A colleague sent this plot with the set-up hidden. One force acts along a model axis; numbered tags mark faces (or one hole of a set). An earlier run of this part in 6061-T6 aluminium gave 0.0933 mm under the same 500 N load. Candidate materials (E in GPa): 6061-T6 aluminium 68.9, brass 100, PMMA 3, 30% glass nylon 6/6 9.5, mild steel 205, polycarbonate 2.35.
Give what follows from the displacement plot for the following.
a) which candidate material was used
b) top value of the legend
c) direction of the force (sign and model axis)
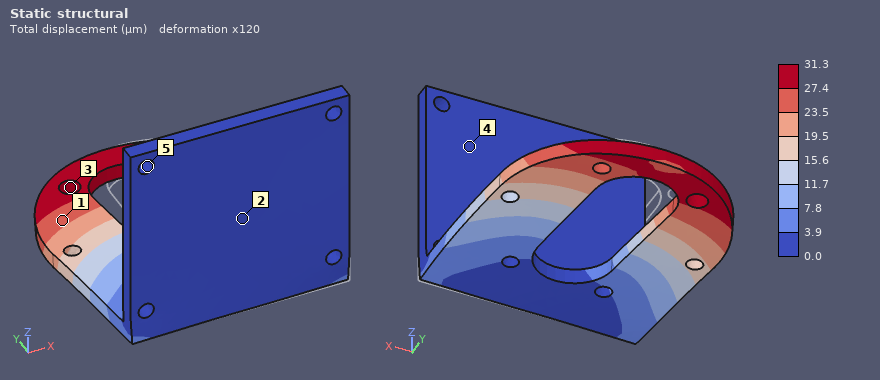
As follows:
mild steel
31.3 µm
-X
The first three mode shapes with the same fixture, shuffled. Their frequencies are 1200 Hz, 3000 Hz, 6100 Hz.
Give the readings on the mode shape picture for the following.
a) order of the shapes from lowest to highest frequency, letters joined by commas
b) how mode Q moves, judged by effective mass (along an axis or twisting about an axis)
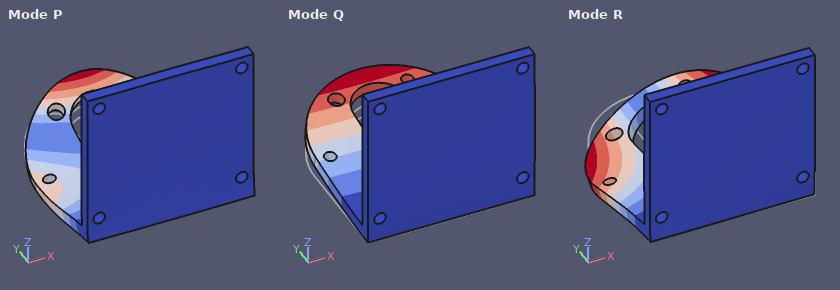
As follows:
Q, R, P
along Z
